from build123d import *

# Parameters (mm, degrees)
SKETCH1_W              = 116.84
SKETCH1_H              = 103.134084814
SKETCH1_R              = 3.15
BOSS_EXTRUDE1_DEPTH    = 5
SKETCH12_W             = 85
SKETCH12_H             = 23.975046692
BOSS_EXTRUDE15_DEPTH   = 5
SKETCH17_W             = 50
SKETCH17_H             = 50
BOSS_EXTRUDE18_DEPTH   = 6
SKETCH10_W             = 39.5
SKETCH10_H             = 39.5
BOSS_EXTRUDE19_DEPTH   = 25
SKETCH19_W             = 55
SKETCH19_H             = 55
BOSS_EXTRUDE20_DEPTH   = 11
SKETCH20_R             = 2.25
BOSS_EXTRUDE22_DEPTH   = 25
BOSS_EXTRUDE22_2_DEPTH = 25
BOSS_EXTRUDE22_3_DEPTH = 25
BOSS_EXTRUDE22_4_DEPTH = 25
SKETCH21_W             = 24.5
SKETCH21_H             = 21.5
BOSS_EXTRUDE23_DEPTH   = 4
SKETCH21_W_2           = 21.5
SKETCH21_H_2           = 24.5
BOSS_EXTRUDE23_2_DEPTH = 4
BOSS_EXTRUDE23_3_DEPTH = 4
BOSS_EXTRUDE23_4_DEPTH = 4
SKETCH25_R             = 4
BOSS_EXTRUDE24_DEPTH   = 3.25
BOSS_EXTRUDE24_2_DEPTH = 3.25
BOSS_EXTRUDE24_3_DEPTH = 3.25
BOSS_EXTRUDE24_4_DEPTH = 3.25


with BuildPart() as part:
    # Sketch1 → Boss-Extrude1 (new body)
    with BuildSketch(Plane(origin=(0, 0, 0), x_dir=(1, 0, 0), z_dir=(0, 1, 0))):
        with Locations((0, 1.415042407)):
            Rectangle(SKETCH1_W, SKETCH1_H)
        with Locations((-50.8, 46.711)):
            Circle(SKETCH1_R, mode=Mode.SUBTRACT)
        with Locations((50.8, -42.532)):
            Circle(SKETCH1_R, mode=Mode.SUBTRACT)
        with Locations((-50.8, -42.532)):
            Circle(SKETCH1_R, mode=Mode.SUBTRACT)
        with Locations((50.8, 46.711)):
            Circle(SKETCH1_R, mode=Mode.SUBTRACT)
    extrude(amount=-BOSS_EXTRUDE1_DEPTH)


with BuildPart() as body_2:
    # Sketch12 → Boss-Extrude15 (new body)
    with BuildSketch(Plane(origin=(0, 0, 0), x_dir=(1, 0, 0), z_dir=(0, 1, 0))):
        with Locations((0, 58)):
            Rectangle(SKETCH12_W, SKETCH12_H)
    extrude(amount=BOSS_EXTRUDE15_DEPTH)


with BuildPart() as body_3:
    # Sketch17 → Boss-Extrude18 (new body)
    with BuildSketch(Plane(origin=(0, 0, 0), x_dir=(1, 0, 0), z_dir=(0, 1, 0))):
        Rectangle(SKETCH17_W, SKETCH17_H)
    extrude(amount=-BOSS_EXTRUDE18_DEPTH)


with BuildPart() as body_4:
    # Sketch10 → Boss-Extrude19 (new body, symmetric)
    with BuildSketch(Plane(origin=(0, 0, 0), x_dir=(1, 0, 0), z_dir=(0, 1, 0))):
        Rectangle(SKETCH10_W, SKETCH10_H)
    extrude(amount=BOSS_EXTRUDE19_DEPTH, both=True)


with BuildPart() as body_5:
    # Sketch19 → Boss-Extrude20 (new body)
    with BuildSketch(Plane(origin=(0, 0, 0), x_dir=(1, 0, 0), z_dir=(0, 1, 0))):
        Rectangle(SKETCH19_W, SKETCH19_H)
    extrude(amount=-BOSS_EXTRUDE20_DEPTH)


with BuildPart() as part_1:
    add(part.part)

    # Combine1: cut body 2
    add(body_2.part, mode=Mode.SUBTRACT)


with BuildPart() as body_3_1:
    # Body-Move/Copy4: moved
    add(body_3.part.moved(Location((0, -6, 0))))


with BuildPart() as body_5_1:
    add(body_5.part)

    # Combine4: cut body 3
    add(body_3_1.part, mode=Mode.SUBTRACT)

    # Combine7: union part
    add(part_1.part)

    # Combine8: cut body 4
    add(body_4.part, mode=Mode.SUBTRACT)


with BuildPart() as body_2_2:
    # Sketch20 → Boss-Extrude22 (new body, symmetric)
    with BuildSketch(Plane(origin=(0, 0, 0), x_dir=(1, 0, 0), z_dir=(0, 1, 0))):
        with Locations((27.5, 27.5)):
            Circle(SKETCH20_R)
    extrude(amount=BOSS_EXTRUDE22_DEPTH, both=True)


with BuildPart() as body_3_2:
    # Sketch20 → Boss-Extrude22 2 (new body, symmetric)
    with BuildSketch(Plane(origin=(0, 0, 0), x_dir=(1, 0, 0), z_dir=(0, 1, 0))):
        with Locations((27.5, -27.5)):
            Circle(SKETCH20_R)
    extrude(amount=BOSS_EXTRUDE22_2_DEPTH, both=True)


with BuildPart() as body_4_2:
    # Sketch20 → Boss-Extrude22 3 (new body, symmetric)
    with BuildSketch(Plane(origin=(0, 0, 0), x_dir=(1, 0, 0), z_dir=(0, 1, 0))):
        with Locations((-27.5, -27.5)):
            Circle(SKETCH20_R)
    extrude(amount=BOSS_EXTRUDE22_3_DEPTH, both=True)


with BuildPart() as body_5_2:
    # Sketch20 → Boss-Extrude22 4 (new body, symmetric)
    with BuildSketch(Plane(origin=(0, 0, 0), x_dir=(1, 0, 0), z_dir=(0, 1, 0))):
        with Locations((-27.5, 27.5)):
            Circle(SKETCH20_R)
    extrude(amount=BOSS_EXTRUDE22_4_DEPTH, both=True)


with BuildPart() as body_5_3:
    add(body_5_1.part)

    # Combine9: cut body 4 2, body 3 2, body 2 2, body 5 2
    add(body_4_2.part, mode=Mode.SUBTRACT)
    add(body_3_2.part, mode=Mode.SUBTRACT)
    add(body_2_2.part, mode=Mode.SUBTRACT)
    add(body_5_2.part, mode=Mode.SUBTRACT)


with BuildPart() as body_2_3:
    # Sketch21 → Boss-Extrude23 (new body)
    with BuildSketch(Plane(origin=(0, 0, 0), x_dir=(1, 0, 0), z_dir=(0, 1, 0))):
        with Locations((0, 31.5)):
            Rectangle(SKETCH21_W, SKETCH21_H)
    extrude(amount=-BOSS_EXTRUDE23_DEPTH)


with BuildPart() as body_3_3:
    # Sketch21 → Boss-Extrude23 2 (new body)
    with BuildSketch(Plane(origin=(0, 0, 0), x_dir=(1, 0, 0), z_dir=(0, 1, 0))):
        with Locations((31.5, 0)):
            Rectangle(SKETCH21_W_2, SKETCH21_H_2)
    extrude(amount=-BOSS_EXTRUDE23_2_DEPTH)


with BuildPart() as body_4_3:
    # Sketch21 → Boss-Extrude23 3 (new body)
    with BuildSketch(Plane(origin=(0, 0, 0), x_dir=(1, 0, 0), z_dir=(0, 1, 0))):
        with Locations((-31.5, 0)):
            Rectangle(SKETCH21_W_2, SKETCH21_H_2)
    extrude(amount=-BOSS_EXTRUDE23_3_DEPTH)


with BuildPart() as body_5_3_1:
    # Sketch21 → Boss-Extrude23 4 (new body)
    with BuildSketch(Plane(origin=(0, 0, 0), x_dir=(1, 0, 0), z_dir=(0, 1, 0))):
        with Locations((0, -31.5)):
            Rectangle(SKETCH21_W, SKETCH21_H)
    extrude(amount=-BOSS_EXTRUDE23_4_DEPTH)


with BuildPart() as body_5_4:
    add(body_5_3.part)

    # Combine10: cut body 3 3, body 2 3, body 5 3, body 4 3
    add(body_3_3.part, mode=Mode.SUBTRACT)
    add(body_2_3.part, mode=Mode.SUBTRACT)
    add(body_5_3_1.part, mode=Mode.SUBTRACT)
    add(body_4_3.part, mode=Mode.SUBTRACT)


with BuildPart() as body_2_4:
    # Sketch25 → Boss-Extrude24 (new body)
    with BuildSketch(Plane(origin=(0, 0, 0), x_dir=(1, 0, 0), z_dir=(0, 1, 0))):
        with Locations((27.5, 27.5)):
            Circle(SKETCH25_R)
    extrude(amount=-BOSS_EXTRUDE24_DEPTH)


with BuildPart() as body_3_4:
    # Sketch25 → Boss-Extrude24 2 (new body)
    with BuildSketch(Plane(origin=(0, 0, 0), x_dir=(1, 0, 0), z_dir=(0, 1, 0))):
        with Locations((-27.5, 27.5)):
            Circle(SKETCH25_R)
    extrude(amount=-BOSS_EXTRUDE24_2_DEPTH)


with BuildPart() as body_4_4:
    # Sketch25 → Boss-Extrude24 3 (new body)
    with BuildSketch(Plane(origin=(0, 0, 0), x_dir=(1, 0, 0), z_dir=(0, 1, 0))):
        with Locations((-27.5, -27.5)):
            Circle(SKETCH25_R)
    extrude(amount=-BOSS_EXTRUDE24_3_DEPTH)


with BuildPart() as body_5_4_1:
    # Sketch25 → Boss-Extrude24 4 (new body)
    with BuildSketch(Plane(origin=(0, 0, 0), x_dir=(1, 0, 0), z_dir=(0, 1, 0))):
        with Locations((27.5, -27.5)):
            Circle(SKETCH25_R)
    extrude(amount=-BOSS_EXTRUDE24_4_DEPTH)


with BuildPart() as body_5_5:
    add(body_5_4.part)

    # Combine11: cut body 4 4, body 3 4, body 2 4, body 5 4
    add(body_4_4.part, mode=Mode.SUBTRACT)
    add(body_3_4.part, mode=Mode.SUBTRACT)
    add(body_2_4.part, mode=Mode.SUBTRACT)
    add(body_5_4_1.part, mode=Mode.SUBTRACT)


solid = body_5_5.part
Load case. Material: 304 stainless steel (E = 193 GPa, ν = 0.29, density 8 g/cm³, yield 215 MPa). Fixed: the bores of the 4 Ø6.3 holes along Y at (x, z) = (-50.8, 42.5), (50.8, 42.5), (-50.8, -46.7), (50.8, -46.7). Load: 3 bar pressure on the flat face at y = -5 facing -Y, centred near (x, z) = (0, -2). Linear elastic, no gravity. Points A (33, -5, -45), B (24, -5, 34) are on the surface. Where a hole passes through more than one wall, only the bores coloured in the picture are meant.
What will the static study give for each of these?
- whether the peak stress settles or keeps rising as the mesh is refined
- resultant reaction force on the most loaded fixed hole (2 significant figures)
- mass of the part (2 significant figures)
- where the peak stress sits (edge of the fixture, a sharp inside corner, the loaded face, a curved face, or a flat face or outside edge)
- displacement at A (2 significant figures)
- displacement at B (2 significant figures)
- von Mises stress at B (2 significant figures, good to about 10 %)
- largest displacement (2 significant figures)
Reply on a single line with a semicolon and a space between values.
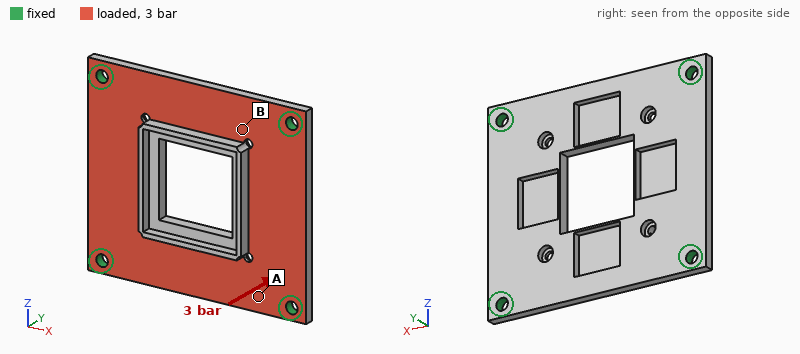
keeps rising; 850 N; 370 g; edge of the fixture; 15 µm; 27 µm; 19 MPa; 47 µm
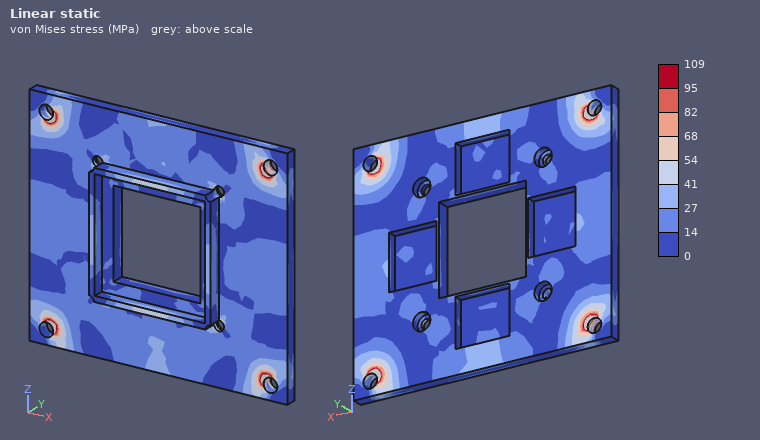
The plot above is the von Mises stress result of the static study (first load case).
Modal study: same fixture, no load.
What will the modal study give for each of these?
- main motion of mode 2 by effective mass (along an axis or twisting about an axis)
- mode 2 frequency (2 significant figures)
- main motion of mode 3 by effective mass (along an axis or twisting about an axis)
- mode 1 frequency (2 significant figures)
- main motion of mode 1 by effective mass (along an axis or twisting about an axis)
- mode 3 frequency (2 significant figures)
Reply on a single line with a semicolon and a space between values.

twisting about X; 3000 Hz; twisting about Z; 2300 Hz; along Y; 3400 Hz
